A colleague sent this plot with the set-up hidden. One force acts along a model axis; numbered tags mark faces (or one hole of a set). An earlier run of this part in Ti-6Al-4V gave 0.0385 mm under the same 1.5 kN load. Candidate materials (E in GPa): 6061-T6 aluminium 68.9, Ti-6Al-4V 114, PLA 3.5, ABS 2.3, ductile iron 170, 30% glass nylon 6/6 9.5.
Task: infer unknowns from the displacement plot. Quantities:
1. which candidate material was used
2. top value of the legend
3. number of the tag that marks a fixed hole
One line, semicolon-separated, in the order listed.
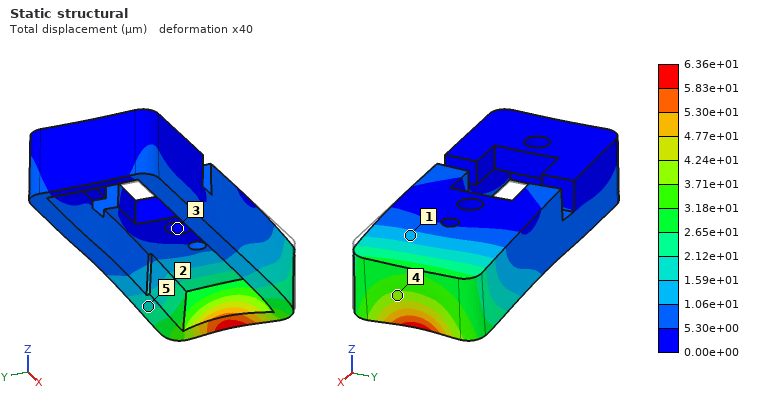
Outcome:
6061-T6 aluminium; 6.36e+01 µm; 3
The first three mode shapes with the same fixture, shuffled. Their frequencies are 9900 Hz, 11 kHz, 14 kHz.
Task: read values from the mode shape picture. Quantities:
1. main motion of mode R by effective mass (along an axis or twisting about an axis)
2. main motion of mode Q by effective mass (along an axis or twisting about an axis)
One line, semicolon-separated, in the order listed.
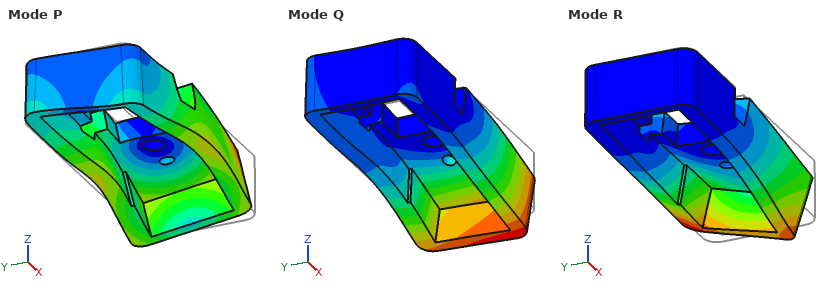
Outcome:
along Y; along Z
